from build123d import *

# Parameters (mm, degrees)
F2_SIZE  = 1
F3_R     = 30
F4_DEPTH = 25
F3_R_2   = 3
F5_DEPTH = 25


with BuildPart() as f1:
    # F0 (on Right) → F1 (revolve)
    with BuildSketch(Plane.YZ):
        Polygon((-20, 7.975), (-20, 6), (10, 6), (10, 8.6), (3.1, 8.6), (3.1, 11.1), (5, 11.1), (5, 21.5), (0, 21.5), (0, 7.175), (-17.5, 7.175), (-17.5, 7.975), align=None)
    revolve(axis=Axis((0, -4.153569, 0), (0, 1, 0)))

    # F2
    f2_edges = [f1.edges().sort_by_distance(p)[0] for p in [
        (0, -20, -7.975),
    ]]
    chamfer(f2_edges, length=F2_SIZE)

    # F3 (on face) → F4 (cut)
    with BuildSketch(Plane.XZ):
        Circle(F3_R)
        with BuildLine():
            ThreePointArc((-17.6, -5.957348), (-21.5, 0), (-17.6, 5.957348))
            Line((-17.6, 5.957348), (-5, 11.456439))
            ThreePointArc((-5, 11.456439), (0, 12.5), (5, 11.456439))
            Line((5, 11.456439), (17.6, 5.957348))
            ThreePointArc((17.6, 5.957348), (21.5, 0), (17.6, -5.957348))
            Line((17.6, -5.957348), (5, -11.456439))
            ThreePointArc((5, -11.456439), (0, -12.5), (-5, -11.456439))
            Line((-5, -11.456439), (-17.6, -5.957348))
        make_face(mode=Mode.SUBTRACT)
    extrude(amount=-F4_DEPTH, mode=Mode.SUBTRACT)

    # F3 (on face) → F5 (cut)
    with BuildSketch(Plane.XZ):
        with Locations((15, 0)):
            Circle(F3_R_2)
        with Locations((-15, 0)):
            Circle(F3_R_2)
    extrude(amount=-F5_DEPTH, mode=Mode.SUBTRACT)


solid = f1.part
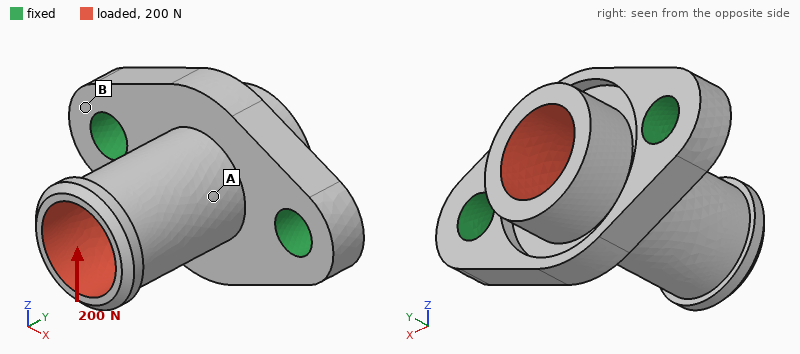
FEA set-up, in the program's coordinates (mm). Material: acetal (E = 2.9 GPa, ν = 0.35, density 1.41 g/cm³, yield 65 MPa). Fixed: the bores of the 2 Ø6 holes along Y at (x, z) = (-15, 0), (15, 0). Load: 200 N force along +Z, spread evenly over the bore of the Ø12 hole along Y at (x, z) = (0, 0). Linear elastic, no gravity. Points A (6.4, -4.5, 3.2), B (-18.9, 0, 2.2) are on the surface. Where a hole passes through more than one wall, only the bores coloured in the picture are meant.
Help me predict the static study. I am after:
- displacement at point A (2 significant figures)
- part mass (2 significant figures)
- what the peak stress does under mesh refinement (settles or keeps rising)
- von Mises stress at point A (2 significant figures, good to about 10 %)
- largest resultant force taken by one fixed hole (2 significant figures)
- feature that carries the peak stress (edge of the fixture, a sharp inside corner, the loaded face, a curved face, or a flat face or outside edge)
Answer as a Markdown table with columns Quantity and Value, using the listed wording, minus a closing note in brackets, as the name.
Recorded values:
| Quantity | Value |
|---|---|
| displacement at point A | 0.11 mm |
| part mass | 6.0 g |
| what the peak stress does under mesh refinement | keeps rising |
| von Mises stress at point A | 6.0 MPa |
| largest resultant force taken by one fixed hole | 100 N |
| feature that carries the peak stress | edge of the fixture |
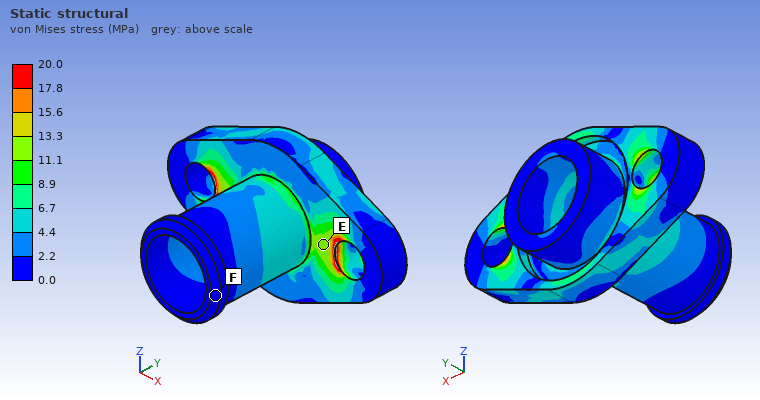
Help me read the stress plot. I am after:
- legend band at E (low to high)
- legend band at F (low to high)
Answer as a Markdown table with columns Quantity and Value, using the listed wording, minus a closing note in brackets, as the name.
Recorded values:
| Quantity | Value |
|---|---|
| legend band at E | 11.1 to 13.3 MPa |
| legend band at F | 0.0 to 2.2 MPa |
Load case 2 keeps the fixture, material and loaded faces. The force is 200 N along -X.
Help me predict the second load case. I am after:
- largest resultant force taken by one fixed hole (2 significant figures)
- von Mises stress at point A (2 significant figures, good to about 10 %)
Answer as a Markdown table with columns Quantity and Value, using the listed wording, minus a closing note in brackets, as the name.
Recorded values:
| Quantity | Value |
|---|---|
| largest resultant force taken by one fixed hole | 120 N |
| von Mises stress at point A | 4.4 MPa |
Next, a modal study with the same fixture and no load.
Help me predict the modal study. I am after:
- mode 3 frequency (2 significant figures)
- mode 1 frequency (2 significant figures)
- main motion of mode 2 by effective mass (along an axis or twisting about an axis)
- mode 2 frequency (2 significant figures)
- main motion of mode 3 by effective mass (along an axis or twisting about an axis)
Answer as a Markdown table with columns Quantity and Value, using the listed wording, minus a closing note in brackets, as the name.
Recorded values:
| Quantity | Value |
|---|---|
| mode 3 frequency | 5300 Hz |
| mode 1 frequency | 2500 Hz |
| main motion of mode 2 by effective mass | along X |
| mode 2 frequency | 4000 Hz |
| main motion of mode 3 by effective mass | along Y |
